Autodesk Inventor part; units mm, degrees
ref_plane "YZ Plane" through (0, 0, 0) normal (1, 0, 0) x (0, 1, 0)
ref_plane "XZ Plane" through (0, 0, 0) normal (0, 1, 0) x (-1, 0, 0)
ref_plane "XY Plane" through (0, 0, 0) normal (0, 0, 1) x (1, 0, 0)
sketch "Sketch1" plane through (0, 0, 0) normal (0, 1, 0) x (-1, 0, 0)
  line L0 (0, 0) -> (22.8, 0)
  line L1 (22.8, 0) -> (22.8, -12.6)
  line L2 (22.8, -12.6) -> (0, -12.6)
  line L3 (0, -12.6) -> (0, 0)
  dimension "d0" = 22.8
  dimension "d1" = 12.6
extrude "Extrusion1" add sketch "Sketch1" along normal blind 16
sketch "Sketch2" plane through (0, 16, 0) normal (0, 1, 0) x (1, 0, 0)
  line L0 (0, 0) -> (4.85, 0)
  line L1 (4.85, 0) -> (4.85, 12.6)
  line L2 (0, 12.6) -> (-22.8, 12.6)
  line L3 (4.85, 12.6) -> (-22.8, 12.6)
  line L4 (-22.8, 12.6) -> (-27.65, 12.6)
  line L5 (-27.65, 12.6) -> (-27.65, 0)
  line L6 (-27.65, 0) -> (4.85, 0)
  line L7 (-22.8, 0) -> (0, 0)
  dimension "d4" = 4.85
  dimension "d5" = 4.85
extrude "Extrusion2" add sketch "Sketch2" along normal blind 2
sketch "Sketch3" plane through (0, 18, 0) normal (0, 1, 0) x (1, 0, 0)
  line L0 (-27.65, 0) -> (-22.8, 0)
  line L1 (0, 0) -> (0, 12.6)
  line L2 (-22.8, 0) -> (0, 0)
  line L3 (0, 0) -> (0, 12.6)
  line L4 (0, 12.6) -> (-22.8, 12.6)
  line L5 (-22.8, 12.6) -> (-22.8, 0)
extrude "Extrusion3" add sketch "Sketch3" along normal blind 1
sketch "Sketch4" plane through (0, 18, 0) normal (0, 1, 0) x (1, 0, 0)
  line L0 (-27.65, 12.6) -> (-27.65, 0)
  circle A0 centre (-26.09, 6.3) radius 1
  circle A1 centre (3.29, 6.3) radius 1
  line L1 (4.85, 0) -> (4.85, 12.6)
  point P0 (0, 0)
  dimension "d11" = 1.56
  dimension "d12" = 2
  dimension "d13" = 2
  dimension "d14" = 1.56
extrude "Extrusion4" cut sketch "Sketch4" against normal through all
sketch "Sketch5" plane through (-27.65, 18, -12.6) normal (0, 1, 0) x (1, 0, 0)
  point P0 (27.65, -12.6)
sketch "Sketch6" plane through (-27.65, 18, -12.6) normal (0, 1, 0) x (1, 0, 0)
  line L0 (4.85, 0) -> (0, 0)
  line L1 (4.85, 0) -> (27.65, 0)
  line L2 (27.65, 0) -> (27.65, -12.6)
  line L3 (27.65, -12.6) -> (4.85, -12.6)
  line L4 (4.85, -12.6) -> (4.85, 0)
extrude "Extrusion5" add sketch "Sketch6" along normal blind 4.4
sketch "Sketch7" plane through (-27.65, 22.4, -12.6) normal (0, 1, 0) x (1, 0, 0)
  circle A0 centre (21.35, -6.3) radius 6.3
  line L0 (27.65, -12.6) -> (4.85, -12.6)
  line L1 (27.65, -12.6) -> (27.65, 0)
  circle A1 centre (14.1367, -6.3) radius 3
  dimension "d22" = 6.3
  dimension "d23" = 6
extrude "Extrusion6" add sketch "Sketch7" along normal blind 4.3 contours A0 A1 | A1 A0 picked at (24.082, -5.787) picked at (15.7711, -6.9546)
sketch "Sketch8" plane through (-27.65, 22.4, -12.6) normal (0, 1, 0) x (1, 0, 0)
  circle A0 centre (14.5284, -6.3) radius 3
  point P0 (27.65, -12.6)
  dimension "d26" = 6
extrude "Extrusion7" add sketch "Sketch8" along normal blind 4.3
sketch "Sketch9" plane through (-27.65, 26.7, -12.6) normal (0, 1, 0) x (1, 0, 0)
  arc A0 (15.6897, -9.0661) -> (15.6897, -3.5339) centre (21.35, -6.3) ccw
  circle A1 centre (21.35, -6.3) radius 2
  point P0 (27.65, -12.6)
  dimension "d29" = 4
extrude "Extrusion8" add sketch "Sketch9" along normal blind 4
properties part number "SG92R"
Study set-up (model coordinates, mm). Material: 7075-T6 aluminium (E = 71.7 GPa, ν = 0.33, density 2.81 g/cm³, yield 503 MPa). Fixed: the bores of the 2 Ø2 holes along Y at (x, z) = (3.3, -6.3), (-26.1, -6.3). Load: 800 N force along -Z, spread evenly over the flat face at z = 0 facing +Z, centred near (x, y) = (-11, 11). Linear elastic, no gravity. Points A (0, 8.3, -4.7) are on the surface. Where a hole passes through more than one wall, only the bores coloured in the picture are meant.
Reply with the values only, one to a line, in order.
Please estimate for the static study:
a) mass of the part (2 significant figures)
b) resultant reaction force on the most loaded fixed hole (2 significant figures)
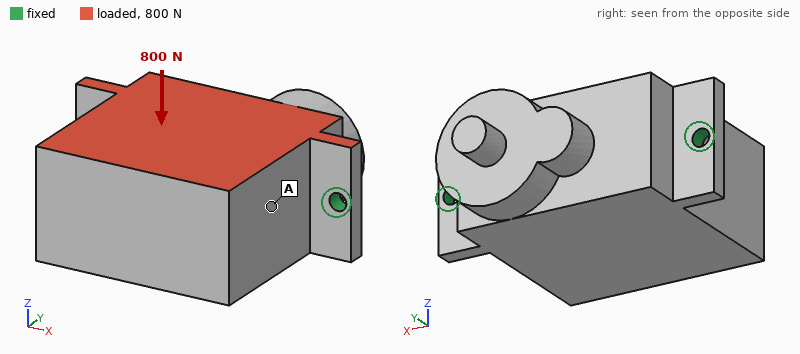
21 g
400 N
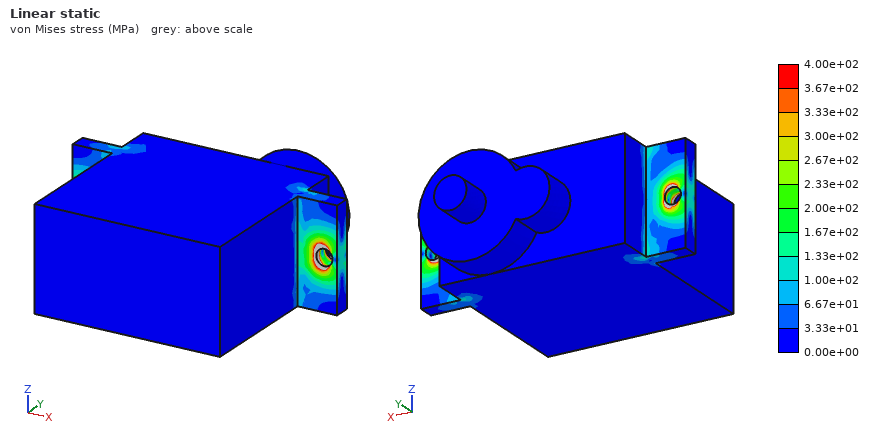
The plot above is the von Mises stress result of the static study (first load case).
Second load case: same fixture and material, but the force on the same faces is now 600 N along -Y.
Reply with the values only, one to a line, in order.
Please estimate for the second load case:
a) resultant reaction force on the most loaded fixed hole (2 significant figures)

300 N
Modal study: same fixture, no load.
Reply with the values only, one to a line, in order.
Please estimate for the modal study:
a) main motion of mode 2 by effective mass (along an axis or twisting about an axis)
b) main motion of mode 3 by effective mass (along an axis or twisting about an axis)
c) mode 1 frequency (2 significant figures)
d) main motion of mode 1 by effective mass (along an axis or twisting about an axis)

along Y
along X
2700 Hz
along Z
